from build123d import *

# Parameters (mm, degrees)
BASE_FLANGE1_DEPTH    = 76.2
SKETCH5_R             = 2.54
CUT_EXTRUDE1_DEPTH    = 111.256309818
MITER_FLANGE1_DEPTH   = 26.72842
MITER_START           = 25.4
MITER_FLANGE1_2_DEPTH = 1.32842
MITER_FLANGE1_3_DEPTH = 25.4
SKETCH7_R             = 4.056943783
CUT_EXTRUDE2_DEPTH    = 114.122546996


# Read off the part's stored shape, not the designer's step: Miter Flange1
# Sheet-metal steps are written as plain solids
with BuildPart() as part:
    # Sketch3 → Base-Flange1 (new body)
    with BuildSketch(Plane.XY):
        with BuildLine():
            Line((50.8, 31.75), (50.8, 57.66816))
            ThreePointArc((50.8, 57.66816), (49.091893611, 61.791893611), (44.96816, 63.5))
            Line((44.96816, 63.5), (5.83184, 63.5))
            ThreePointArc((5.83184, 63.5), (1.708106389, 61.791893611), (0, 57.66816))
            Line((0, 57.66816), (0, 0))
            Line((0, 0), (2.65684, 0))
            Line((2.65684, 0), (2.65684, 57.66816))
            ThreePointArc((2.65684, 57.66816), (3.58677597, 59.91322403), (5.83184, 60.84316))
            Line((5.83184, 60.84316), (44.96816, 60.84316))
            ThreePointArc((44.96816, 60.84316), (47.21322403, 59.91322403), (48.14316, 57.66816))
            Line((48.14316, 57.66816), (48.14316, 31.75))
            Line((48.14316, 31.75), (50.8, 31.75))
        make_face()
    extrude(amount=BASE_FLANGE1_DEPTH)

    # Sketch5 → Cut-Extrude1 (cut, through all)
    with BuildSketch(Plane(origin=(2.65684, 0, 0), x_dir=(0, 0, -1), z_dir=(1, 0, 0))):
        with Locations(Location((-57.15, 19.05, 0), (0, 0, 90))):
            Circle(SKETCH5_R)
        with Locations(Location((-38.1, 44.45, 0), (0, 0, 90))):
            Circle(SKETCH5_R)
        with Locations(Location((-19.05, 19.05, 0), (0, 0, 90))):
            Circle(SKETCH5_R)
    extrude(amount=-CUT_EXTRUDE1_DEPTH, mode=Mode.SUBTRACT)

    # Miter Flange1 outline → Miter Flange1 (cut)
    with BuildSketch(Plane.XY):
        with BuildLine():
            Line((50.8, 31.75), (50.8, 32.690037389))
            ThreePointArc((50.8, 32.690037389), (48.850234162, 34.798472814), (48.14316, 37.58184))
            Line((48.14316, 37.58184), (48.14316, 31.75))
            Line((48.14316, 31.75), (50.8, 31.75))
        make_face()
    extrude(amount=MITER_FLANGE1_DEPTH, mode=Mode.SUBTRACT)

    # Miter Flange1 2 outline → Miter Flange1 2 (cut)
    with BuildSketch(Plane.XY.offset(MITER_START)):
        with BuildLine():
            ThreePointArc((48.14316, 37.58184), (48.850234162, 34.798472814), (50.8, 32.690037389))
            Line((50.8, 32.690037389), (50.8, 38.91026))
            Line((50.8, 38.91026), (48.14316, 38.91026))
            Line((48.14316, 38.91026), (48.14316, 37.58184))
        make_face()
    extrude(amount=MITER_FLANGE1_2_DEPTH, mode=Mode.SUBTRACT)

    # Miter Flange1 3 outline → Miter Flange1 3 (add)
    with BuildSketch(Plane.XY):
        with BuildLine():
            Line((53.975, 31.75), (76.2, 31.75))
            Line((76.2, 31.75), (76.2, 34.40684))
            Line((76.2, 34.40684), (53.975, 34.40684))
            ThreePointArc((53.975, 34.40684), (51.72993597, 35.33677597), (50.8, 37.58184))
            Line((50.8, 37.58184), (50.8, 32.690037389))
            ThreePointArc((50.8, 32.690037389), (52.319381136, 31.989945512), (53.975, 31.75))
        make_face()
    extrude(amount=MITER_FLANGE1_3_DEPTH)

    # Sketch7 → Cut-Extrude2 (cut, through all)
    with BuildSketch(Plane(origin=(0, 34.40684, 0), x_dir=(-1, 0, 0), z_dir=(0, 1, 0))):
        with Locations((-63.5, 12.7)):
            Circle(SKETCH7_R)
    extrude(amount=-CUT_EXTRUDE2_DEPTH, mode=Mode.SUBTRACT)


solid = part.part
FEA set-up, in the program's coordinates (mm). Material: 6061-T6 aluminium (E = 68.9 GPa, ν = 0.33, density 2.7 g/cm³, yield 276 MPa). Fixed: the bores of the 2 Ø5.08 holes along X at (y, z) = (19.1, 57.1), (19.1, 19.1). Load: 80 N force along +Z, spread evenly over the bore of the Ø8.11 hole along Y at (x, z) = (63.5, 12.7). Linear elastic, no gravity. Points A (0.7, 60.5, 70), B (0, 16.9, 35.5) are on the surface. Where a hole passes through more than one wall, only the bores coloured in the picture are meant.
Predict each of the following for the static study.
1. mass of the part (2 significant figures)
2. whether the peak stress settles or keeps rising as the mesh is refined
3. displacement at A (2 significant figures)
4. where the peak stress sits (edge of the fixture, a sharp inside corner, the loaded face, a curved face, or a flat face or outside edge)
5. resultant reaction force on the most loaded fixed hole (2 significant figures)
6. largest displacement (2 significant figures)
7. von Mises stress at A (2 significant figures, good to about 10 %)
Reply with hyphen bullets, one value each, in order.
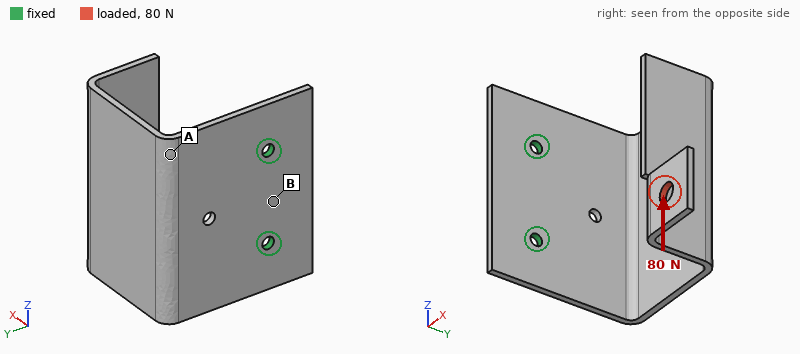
- 78 g
- keeps rising
- 0.31 mm
- edge of the fixture
- 110 N
- 1.2 mm
- 29 MPa
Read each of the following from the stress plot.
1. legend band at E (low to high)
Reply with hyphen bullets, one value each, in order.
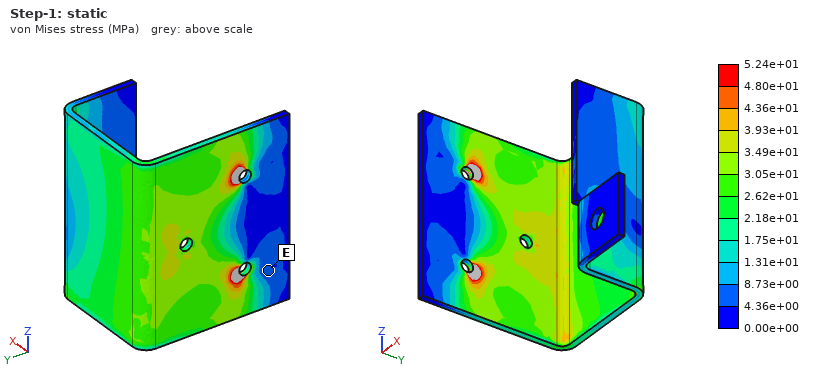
- 4.36e+00 to 8.73e+00 MPa
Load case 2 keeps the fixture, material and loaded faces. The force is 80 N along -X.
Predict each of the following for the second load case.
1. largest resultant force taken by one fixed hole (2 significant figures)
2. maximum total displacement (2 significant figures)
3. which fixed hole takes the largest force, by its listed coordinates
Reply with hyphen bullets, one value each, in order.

- 81 N
- 1.4 mm
- (19.1, 19.1)
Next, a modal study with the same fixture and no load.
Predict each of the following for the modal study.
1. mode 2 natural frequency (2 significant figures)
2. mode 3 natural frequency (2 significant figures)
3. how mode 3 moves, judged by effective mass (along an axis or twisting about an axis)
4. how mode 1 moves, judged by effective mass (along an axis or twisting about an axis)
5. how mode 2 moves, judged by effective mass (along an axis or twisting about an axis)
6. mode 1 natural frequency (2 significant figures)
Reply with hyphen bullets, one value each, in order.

- 340 Hz
- 510 Hz
- along X
- along Y
- along Z
- 210 Hz
